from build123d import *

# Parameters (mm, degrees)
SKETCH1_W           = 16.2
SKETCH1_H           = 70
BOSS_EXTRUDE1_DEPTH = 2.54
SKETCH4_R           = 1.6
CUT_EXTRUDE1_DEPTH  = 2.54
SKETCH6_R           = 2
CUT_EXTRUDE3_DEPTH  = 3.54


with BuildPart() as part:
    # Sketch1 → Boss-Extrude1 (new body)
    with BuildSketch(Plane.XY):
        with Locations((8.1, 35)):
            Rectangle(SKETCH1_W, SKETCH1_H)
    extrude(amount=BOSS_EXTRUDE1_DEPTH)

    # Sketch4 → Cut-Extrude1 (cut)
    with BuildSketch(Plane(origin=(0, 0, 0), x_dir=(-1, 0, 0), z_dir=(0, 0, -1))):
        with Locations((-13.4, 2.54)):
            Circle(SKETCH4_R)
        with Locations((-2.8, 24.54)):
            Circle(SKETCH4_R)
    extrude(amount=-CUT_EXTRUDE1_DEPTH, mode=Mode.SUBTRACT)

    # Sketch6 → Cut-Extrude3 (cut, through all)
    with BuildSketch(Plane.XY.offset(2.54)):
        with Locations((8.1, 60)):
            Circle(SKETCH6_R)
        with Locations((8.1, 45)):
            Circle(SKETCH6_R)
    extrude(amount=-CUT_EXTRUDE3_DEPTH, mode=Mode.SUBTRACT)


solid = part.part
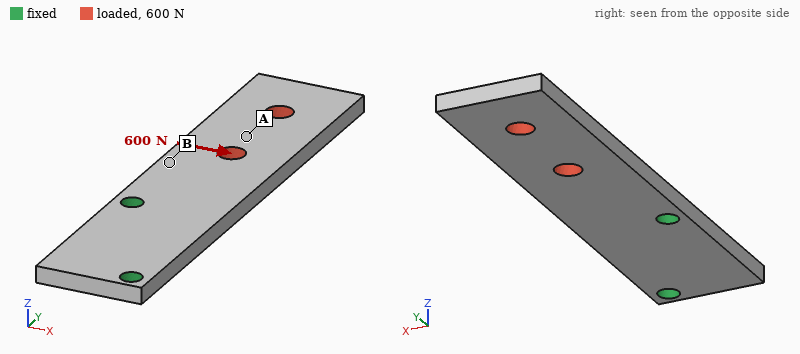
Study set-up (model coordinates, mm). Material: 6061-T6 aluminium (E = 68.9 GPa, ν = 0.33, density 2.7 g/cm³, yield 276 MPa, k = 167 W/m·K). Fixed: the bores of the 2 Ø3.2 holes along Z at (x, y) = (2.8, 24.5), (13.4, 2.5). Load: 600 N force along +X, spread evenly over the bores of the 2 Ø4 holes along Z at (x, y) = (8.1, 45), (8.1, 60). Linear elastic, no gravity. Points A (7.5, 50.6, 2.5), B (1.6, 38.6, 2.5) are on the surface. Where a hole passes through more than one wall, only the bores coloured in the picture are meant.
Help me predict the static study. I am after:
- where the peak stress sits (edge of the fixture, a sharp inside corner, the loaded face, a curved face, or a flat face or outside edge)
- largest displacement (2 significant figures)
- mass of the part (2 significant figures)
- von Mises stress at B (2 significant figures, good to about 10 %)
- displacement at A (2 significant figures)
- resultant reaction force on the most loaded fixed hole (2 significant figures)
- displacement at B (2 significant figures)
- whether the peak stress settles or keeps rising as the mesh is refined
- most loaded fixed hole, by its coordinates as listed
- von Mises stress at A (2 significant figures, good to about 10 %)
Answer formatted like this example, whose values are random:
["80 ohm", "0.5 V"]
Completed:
["edge of the fixture", "0.24 mm", "7.5 g", "62 MPa", "0.12 mm", "1.2 kN", "0.057 mm", "keeps rising", "(2.8, 24.5)", "28 MPa"]
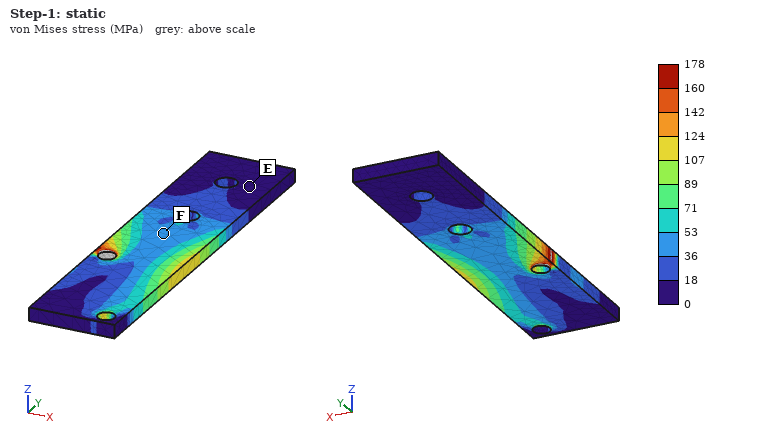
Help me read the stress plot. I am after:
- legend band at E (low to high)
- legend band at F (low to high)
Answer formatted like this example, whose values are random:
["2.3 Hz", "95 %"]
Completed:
["0 to 18 MPa", "36 to 53 MPa"]
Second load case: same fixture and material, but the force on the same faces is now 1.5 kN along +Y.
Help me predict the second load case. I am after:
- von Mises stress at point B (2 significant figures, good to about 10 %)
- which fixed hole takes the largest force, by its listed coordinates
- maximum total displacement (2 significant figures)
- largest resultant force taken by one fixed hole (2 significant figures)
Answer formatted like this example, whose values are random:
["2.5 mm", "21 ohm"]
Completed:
["37 MPa", "(2.8, 24.5)", "47 µm", "1.1 kN"]
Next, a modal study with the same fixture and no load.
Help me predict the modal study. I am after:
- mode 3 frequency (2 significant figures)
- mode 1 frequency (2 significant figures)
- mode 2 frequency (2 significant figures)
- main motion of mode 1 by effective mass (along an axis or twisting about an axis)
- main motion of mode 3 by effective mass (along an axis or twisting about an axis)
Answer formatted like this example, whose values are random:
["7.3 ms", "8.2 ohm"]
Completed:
["4900 Hz", "990 Hz", "4600 Hz", "along Z", "along X"]
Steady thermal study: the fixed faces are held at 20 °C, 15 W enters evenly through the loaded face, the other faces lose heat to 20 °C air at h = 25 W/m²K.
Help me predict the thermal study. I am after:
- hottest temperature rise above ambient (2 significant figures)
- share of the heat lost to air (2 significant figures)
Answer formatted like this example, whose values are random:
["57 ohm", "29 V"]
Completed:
["64 K", "12 %"]
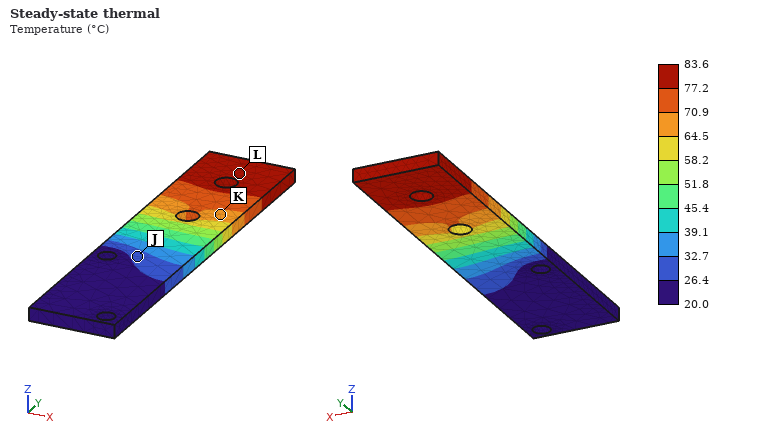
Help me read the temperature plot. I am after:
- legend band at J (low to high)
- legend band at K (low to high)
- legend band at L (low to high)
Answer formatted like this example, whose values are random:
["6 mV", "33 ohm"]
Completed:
["26.4 to 32.7 °C", "64.5 to 70.9 °C", "77.2 to 83.6 °C"]
